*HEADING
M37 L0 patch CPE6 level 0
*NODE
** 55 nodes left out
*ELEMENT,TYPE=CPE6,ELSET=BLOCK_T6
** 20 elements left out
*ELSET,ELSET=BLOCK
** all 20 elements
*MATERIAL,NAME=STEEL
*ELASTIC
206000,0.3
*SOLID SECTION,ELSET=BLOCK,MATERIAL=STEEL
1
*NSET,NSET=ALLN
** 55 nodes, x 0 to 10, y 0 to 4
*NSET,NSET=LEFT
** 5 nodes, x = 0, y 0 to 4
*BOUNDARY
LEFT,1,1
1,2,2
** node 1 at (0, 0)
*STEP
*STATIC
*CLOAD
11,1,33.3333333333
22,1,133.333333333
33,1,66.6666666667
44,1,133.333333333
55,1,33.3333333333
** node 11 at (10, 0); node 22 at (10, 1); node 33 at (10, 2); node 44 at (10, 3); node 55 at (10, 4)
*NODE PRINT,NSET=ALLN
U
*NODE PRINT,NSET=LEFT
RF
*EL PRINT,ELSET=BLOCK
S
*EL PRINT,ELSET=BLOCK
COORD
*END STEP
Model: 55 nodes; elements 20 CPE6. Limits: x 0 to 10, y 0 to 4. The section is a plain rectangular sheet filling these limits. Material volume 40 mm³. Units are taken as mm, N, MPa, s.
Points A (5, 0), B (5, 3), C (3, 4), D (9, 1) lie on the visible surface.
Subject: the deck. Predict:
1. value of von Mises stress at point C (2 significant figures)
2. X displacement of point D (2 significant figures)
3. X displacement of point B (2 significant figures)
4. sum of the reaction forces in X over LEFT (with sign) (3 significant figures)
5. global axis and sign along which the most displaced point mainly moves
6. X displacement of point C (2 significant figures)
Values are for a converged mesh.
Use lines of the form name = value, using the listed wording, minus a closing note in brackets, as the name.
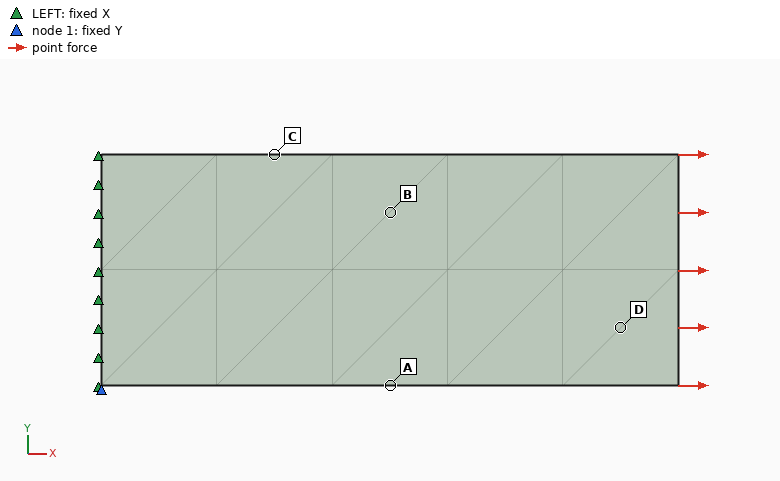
value of von Mises stress at point C = 89 MPa
X displacement of point D = 0.0040 mm
X displacement of point B = 0.0022 mm
sum of the reaction forces in X over LEFT (with sign) = -400 N
global axis and sign along which the most displaced point mainly moves = +X
X displacement of point C = 0.0013 mm
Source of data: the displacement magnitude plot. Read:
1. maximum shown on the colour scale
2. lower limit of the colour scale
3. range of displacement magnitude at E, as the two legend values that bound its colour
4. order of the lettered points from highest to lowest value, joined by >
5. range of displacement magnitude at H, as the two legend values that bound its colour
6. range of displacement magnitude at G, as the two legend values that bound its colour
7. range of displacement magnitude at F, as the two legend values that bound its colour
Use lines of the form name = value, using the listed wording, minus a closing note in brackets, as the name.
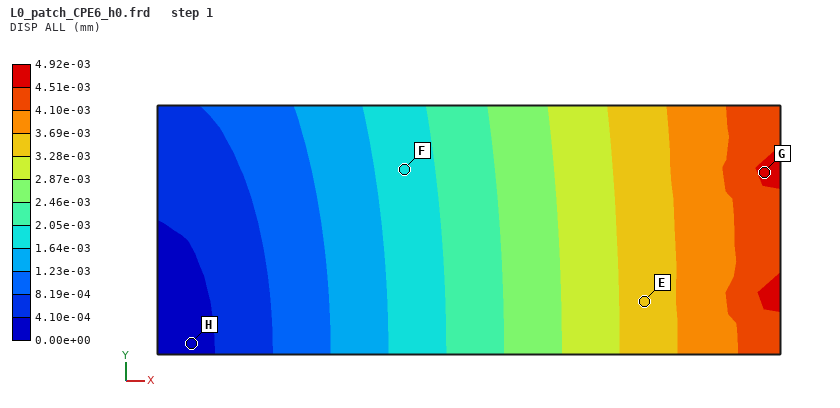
maximum shown on the colour scale = 4.92e-03 mm
lower limit of the colour scale = 0.00e+00 mm
range of displacement magnitude at E, as the two legend values that bound its colour = 3.28e-03 to 3.69e-03 mm
order of the lettered points from highest to lowest value, joined by > = G > E > F > H
range of displacement magnitude at H, as the two legend values that bound its colour = 0.00e+00 to 4.10e-04 mm
range of displacement magnitude at G, as the two legend values that bound its colour = 4.51e-03 to 4.92e-03 mm
range of displacement magnitude at F, as the two legend values that bound its colour = 1.64e-03 to 2.05e-03 mm
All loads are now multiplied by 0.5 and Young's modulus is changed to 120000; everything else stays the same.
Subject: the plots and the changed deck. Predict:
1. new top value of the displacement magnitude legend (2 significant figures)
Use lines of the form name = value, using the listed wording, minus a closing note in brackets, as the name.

new top value of the displacement magnitude legend = 0.0042 mm
